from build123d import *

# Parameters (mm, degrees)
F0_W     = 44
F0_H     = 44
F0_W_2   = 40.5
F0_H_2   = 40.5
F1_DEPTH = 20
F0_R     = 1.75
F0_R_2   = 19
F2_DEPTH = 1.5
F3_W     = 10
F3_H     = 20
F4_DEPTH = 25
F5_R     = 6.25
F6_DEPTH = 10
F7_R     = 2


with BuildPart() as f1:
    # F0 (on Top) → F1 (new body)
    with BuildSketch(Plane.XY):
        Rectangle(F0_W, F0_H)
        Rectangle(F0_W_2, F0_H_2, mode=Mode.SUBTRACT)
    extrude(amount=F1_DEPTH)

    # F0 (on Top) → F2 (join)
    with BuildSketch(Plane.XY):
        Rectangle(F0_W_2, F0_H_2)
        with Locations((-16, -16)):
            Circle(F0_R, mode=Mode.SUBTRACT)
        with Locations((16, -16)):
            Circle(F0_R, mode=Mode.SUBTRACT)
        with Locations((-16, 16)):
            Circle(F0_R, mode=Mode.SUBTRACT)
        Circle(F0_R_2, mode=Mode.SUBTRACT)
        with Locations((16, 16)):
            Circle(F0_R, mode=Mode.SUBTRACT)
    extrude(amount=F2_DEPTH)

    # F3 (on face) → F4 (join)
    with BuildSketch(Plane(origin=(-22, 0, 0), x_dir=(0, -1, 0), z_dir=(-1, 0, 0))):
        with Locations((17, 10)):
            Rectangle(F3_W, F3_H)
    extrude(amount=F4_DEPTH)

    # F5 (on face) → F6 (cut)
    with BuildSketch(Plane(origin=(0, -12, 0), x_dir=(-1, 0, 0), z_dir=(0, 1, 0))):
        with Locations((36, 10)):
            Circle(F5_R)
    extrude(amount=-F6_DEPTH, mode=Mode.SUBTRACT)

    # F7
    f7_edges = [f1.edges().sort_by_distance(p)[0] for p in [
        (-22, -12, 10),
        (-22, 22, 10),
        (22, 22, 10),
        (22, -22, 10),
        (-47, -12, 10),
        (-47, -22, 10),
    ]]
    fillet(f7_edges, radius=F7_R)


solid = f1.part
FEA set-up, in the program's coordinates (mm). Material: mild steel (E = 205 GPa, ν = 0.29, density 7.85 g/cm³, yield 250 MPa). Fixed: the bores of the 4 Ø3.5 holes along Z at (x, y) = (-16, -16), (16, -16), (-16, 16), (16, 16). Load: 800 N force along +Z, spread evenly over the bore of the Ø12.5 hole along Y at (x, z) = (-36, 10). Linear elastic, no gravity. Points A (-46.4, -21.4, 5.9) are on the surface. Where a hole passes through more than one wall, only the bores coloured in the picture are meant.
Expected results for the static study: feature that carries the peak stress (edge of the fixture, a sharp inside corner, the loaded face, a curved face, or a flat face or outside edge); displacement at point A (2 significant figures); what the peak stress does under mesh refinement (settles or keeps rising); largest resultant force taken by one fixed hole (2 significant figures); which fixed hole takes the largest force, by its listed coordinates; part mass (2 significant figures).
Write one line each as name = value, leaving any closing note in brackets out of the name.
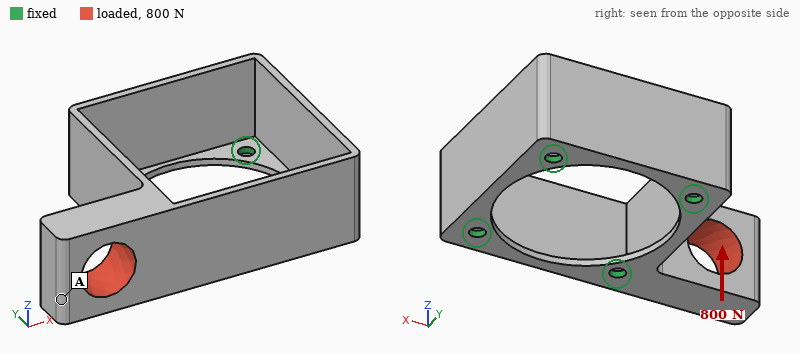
feature that carries the peak stress = edge of the fixture
displacement at point A = 61 µm
what the peak stress does under mesh refinement = keeps rising
largest resultant force taken by one fixed hole = 1.3 kN
which fixed hole takes the largest force, by its listed coordinates = (-16, -16)
part mass = 81 g
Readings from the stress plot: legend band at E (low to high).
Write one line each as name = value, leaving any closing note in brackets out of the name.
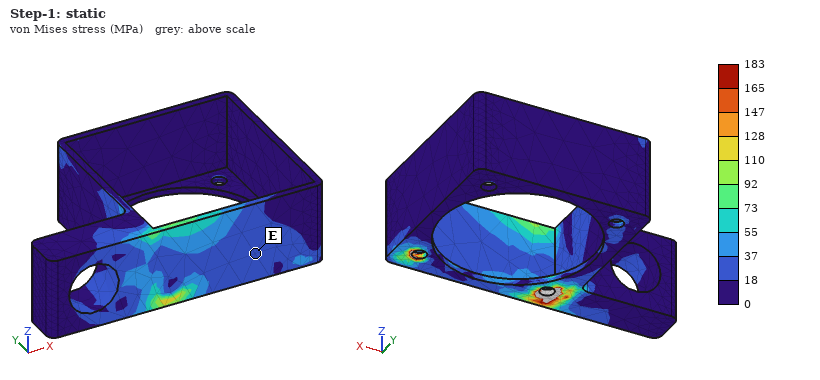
legend band at E = 18 to 37 MPa
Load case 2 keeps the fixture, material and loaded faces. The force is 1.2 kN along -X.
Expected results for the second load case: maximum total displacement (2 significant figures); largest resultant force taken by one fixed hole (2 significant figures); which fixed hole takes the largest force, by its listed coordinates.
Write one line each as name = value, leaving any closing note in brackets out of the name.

maximum total displacement = 37 µm
largest resultant force taken by one fixed hole = 910 N
which fixed hole takes the largest force, by its listed coordinates = (-16, -16)
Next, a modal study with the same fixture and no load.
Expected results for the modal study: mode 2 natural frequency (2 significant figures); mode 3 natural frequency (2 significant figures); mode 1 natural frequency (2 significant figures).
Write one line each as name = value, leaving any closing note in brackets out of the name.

mode 2 natural frequency = 4600 Hz
mode 3 natural frequency = 5000 Hz
mode 1 natural frequency = 3100 Hz
